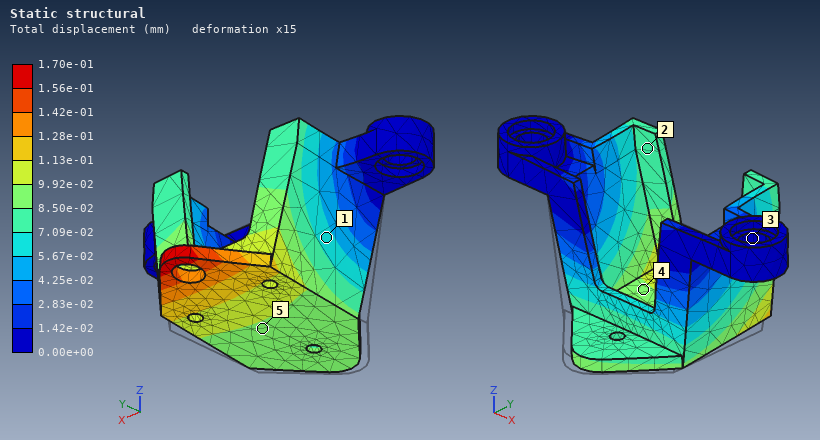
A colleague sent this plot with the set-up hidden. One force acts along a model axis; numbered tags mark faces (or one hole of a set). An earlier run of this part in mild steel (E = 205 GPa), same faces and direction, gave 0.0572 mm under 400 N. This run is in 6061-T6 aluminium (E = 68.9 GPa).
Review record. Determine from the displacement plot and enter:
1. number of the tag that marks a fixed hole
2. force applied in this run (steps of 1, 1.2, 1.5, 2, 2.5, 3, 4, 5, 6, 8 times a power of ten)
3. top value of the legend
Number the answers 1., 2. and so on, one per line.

1. 3
2. 400 N
3. 1.70e-01 mm
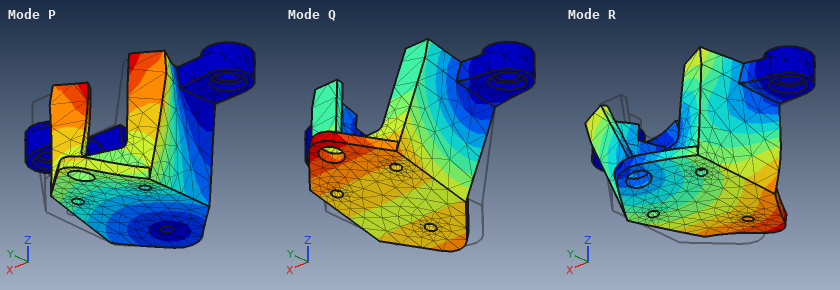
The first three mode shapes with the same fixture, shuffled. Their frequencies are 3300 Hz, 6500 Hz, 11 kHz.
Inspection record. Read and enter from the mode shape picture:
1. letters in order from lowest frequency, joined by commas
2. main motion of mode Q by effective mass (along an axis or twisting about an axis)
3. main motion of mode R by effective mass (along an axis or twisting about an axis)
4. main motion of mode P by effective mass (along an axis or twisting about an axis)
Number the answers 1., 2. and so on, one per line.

1. Q, P, R
2. along Y
3. along X
4. along X
